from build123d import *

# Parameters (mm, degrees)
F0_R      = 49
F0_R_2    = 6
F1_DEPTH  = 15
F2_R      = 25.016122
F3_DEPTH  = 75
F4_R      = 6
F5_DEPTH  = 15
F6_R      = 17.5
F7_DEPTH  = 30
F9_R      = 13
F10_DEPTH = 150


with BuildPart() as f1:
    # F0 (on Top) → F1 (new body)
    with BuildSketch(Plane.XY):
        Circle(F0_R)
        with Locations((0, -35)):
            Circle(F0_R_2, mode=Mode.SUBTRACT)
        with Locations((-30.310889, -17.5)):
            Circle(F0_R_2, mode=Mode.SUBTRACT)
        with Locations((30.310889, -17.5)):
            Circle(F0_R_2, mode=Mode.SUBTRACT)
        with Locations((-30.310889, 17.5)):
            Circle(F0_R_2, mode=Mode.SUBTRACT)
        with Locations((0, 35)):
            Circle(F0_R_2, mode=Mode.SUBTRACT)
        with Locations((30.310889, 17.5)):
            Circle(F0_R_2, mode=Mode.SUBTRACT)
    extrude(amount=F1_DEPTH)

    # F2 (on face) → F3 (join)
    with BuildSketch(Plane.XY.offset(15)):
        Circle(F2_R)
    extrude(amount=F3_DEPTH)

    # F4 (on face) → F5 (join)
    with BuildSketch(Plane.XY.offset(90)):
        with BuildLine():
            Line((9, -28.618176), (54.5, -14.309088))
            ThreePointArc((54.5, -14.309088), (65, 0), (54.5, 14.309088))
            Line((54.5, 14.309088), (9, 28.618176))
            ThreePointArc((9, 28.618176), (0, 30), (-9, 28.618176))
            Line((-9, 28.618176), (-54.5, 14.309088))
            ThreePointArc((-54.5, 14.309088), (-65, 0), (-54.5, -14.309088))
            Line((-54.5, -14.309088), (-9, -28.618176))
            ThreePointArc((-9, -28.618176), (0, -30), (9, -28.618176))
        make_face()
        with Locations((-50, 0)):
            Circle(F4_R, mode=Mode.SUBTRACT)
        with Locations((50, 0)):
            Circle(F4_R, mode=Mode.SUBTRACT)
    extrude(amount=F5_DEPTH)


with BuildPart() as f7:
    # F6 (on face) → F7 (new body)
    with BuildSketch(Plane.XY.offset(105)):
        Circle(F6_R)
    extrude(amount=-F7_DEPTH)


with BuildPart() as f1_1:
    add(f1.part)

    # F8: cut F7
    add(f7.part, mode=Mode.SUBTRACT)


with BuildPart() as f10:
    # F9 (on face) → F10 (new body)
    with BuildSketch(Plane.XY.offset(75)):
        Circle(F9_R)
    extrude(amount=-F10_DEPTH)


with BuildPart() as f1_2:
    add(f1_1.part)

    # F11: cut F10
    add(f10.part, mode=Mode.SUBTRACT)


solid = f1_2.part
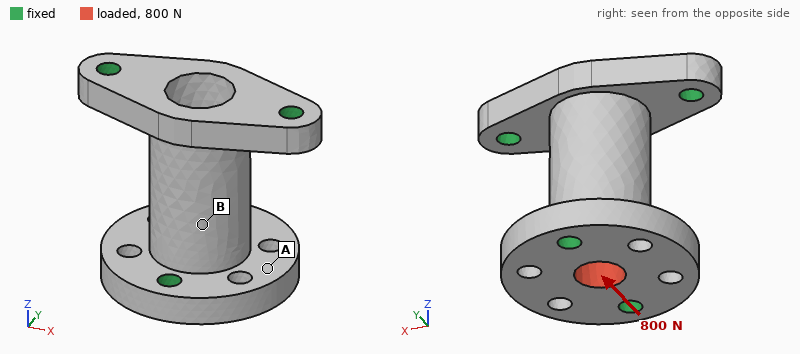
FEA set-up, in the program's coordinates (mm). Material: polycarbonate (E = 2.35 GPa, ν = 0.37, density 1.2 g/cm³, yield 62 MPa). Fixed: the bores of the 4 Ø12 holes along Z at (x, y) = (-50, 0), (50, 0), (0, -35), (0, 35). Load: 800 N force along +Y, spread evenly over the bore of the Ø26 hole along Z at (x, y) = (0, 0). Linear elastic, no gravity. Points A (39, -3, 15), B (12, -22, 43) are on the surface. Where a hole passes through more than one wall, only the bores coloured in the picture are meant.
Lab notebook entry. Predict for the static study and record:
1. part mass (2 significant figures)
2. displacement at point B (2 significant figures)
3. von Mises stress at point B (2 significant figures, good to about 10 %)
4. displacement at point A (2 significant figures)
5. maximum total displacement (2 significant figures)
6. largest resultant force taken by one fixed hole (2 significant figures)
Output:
310 g
20 µm
0.42 MPa
5.8 µm
24 µm
330 N
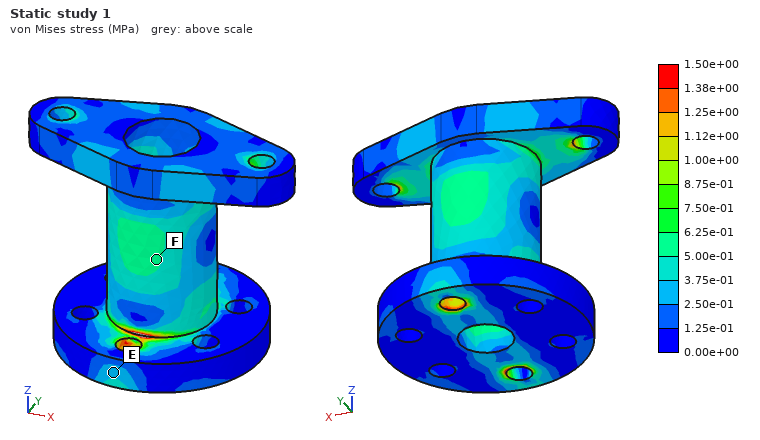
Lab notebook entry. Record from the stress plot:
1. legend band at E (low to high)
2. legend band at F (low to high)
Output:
2.50e-01 to 3.75e-01 MPa
5.00e-01 to 6.25e-01 MPa
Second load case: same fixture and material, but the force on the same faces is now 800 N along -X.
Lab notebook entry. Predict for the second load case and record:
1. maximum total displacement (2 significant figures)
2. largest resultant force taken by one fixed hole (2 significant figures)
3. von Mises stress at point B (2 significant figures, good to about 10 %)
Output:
25 µm
260 N
0.31 MPa
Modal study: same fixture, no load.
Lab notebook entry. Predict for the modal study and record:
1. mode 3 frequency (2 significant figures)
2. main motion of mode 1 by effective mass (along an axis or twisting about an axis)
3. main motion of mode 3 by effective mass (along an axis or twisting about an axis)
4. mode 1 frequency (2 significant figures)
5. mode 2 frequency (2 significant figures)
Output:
2400 Hz
along Z
along Y
1900 Hz
2100 Hz
